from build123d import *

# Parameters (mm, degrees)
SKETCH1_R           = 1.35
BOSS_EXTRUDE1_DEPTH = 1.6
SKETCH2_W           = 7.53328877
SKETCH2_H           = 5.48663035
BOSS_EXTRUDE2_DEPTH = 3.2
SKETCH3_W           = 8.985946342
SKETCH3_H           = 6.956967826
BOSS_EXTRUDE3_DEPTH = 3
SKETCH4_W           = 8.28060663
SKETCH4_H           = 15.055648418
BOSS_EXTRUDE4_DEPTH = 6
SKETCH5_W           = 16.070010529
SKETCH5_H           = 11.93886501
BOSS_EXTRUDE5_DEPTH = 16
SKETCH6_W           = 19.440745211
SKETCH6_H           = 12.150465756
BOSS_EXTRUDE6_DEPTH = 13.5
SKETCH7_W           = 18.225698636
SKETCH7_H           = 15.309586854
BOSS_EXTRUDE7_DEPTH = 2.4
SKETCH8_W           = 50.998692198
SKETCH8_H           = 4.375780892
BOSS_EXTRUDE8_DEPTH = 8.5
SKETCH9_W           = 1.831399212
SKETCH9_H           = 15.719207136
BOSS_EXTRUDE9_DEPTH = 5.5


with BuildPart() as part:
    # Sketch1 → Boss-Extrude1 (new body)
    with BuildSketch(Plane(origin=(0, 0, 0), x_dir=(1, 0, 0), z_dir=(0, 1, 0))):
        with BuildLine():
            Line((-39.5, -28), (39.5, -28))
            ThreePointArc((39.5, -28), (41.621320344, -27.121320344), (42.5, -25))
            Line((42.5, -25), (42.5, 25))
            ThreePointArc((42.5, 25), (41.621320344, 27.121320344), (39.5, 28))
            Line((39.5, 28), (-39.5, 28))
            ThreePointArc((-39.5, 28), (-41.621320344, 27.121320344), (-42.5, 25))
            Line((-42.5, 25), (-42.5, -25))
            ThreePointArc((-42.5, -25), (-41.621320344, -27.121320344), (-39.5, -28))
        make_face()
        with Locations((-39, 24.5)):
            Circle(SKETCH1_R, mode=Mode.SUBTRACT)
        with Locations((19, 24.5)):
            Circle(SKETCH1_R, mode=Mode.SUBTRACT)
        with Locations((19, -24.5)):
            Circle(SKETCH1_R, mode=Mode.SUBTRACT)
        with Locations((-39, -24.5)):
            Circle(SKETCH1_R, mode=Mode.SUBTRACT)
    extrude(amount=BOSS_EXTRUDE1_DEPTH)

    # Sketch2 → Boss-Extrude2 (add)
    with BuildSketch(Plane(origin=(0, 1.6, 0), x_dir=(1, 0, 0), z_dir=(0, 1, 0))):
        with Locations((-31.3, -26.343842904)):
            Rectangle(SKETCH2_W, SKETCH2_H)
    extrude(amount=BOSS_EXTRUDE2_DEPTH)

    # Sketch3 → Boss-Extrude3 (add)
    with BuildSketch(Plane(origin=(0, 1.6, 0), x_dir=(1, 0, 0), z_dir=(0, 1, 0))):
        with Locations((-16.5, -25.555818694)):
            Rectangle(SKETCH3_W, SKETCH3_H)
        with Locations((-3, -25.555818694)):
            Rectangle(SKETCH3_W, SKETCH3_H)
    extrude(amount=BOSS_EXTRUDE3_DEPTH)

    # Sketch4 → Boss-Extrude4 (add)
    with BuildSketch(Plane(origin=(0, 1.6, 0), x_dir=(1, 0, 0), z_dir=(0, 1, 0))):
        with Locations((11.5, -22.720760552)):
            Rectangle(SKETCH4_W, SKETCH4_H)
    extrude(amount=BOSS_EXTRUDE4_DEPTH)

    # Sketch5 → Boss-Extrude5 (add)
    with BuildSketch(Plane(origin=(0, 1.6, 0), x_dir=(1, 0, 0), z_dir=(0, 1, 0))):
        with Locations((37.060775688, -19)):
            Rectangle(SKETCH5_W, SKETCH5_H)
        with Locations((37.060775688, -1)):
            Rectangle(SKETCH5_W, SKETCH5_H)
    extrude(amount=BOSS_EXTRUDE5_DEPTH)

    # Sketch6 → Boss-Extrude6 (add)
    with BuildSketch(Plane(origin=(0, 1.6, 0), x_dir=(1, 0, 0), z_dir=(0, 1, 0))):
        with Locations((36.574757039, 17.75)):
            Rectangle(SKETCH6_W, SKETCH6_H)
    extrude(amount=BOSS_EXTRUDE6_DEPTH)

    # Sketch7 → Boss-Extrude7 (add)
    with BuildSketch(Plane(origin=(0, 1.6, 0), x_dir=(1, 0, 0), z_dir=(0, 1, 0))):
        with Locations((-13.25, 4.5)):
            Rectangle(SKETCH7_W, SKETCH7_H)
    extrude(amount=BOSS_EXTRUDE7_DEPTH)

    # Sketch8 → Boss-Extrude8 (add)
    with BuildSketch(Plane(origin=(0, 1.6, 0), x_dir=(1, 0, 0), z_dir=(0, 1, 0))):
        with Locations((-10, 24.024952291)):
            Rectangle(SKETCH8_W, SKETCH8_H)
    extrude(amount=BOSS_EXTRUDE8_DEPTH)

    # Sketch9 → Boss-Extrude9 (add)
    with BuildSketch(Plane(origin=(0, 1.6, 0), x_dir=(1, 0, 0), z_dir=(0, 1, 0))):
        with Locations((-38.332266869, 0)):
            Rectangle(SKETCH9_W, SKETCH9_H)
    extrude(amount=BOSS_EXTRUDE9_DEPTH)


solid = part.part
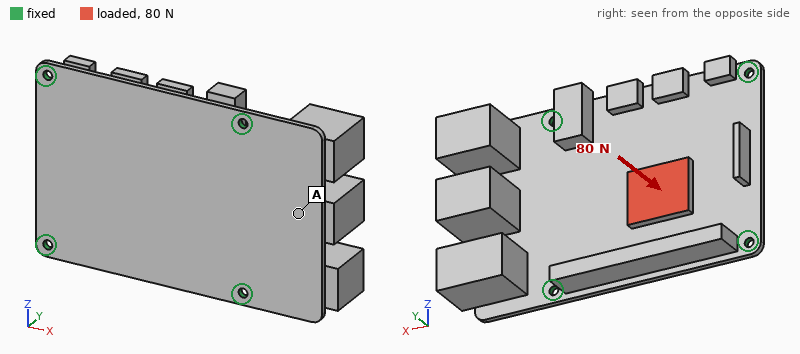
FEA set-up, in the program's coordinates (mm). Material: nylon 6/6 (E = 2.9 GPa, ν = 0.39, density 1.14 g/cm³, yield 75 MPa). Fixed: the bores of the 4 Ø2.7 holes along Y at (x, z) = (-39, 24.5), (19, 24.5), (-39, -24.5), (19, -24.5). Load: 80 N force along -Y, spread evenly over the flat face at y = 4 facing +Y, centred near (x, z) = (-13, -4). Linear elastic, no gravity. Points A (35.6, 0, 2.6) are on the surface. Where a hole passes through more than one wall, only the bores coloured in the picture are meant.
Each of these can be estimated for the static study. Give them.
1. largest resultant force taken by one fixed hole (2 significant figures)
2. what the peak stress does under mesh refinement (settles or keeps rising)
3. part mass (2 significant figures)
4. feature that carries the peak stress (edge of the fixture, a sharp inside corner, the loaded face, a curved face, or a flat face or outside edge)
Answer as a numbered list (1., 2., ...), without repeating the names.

1. 43 N
2. keeps rising
3. 24 g
4. edge of the fixture
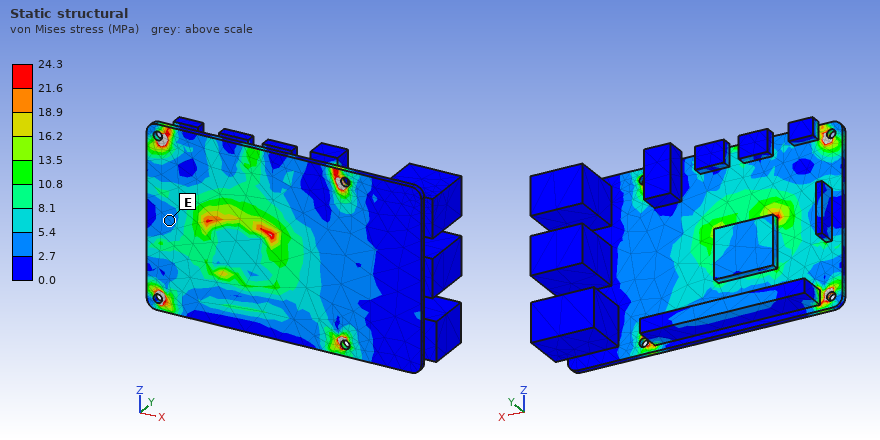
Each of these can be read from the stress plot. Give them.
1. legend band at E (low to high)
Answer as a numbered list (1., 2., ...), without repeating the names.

1. 2.7 to 5.4 MPa
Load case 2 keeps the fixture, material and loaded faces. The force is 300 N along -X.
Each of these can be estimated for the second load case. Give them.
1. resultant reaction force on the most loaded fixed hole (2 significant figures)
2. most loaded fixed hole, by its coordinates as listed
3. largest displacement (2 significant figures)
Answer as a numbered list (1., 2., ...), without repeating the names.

1. 100 N
2. (19, -24.5)
3. 0.34 mm
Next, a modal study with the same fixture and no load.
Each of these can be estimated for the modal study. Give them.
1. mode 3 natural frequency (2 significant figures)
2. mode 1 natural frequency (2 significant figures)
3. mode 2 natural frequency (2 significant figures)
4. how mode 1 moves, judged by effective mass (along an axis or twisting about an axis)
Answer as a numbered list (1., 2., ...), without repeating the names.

1. 590 Hz
2. 180 Hz
3. 520 Hz
4. along Y
